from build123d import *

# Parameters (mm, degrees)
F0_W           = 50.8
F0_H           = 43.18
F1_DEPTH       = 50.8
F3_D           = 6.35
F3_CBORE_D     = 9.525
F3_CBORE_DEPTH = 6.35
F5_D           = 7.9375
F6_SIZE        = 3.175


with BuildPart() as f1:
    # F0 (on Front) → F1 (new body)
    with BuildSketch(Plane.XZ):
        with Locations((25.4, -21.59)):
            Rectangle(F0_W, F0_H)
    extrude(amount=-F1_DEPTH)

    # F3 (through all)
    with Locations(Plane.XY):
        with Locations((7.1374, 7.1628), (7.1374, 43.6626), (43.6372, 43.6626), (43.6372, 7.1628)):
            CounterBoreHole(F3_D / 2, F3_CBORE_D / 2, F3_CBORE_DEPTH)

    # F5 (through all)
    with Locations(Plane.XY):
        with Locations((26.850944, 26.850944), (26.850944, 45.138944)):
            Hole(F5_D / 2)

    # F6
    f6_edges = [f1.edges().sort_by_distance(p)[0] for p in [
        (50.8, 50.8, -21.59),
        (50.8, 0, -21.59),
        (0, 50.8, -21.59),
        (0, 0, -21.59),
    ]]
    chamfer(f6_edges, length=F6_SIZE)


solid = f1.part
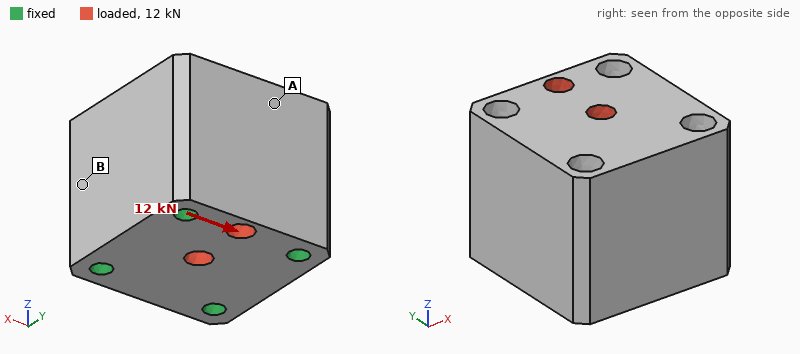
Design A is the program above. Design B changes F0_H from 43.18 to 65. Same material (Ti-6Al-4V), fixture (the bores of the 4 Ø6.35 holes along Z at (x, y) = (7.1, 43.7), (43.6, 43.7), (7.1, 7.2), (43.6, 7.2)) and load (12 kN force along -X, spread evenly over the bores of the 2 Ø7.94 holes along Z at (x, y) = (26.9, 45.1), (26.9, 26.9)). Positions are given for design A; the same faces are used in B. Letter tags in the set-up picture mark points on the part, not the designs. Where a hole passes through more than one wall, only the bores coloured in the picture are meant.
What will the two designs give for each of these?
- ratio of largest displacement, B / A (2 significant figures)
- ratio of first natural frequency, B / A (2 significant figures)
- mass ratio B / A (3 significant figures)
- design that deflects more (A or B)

1.6
0.71
1.49
B
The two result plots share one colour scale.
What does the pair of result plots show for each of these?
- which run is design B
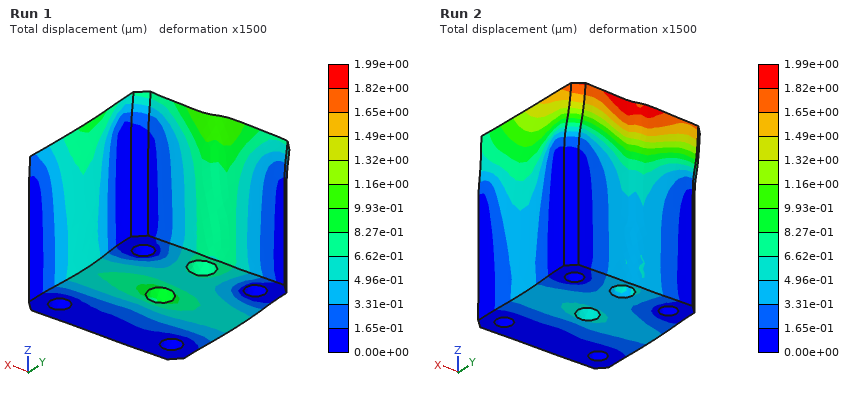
Run 2
